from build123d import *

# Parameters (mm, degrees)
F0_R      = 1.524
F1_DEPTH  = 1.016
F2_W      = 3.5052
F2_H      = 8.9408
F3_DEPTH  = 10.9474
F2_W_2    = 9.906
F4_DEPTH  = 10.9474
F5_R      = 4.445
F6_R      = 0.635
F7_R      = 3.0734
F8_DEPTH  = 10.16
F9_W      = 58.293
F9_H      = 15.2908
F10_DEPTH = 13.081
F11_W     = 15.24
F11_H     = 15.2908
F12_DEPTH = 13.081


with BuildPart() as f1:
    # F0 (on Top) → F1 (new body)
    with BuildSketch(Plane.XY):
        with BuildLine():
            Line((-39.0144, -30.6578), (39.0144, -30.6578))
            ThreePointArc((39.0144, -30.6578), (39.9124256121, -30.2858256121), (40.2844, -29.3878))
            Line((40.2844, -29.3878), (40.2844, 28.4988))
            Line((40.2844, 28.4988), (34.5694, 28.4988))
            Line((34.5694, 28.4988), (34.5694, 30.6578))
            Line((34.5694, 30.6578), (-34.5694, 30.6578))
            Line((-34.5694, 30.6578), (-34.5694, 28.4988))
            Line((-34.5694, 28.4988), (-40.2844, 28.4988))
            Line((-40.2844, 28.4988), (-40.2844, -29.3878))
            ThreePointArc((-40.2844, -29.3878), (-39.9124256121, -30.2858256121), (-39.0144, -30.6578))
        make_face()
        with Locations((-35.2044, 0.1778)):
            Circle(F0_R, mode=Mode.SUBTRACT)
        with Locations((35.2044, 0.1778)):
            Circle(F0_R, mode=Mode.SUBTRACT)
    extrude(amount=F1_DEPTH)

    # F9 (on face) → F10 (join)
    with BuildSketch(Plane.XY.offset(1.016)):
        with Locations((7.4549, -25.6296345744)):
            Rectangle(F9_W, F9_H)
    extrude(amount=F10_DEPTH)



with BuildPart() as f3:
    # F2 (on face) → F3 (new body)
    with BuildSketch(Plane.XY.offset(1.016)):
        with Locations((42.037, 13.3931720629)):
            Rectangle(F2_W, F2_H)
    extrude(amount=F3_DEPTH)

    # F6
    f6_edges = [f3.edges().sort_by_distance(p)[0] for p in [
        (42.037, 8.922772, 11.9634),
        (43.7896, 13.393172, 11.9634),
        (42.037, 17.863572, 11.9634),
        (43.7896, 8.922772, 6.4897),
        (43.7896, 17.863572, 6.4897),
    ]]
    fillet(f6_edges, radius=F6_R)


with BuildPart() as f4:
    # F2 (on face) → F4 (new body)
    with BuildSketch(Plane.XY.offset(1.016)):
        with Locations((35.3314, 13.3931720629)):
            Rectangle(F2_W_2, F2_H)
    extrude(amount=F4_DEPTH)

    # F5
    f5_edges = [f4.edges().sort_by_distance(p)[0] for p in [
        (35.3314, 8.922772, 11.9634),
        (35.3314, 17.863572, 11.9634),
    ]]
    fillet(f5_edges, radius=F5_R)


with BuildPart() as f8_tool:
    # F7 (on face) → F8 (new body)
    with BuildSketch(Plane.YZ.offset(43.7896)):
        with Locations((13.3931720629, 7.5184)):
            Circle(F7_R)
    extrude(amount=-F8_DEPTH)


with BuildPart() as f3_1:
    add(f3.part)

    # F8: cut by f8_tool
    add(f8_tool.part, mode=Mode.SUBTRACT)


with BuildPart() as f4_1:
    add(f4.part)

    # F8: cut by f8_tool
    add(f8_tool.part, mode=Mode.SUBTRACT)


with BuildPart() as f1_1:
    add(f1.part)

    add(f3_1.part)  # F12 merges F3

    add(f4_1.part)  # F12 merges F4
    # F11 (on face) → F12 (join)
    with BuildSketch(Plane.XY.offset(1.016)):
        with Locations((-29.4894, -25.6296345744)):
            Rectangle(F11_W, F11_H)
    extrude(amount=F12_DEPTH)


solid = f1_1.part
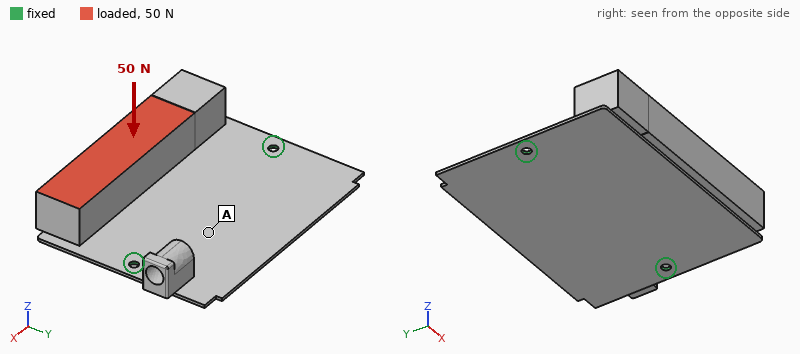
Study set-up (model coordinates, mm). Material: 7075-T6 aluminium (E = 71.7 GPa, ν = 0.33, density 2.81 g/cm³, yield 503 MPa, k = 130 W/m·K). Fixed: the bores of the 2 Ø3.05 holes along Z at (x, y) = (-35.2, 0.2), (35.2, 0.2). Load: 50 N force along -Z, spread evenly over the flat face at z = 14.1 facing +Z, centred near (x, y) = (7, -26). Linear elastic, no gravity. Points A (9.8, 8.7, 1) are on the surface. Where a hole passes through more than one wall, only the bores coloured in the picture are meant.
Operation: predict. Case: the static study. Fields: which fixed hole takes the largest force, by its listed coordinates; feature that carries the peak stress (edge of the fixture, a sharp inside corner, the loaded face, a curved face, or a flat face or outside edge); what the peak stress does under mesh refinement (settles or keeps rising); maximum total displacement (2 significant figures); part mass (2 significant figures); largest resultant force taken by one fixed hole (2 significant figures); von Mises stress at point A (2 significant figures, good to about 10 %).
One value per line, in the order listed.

(35.2, 0.2)
edge of the fixture
keeps rising
1.2 mm
58 g
30 N
17 MPa
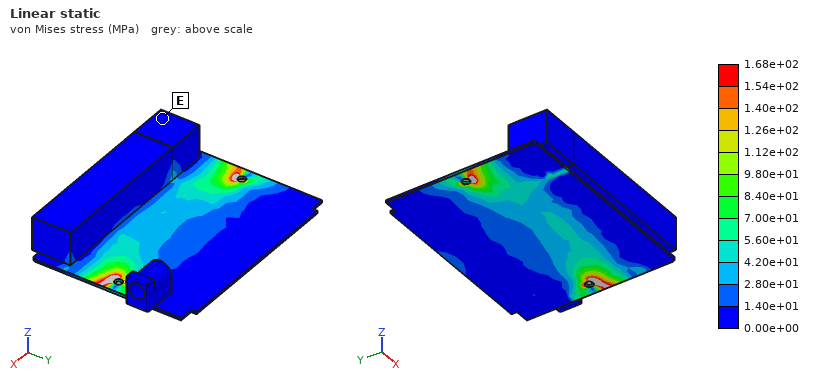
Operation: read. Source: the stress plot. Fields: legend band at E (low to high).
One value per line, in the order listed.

0.00e+00 to 1.40e+01 MPa
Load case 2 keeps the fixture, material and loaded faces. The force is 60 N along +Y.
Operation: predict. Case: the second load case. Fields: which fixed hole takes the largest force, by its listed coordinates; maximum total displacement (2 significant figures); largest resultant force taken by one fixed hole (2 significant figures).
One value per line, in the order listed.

(35.2, 0.2)
1.0 mm
36 N
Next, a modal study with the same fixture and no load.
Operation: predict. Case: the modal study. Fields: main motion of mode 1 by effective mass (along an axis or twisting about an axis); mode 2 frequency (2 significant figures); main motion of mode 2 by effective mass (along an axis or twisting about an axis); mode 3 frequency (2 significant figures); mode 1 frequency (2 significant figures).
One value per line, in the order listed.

along Z
630 Hz
along Z
760 Hz
170 Hz
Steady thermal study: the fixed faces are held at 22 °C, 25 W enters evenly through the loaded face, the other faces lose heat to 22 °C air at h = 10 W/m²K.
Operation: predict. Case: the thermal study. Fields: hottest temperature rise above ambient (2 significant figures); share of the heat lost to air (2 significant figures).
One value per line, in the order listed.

74 K
23 %
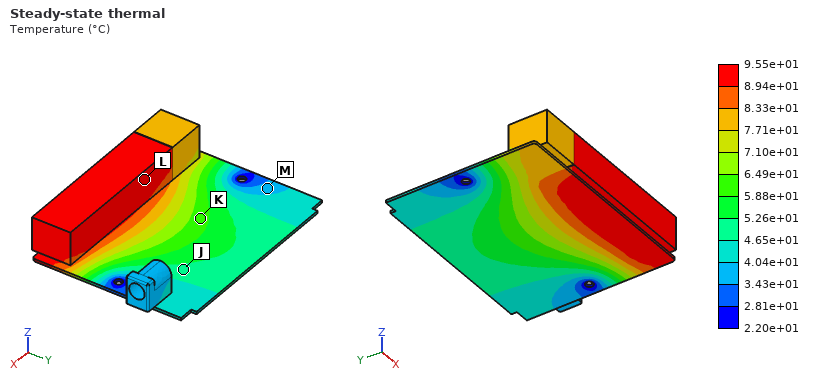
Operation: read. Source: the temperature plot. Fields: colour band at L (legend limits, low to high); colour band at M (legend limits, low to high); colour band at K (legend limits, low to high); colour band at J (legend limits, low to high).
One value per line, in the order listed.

8.94e+01 to 9.55e+01 °C
3.43e+01 to 4.04e+01 °C
5.88e+01 to 6.49e+01 °C
4.65e+01 to 5.26e+01 °C
